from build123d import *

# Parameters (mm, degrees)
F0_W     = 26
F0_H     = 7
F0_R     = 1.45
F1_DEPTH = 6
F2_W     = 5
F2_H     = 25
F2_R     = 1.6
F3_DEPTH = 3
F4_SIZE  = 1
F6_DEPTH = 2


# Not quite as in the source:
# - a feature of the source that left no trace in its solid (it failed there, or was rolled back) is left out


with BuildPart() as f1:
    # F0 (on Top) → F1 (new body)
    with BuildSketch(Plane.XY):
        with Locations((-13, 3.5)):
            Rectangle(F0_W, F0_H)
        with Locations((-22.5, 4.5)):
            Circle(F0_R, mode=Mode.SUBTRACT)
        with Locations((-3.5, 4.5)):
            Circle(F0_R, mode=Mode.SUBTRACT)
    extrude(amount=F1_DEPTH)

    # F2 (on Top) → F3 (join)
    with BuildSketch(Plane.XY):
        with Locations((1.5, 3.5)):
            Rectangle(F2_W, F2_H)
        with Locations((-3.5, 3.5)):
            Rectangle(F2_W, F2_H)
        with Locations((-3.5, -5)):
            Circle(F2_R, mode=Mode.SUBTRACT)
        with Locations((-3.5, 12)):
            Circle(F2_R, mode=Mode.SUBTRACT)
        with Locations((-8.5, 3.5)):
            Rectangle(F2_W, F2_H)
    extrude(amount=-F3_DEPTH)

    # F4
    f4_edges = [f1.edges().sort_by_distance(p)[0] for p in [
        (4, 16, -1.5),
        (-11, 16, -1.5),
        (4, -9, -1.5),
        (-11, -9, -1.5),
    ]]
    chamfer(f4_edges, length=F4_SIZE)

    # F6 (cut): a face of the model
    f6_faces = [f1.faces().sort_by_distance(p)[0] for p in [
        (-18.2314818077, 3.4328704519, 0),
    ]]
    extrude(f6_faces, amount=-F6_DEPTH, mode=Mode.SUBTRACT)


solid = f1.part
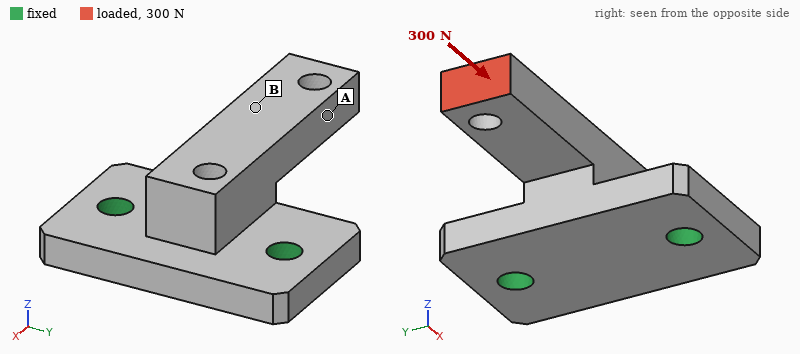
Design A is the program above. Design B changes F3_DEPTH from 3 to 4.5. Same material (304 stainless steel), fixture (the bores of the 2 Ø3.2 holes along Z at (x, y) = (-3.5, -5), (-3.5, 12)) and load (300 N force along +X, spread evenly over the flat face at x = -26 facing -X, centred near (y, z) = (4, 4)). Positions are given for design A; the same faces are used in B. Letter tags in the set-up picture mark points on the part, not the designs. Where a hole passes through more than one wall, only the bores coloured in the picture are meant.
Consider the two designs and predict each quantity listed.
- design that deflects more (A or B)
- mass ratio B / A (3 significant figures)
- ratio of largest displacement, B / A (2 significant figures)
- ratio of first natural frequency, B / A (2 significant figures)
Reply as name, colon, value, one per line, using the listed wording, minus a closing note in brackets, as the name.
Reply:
design that deflects more: A
mass ratio B / A: 1.28
ratio of largest displacement, B / A: 0.57
ratio of first natural frequency, B / A: 1.2
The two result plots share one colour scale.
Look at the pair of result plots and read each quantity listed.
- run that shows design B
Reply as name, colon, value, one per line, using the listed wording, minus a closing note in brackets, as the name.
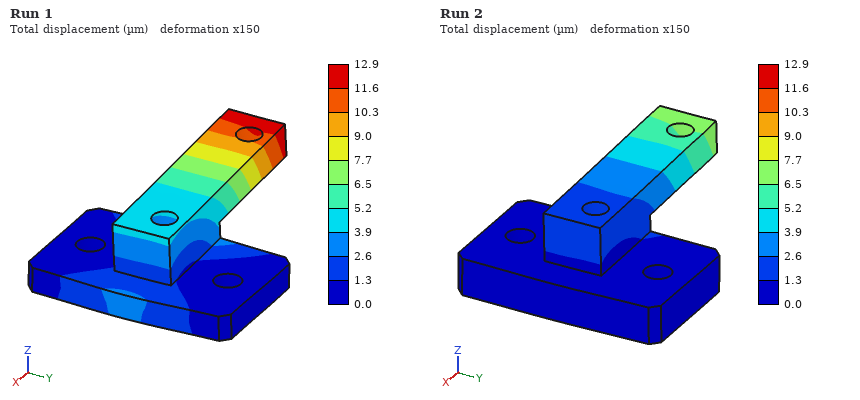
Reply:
run that shows design B: Run 2
